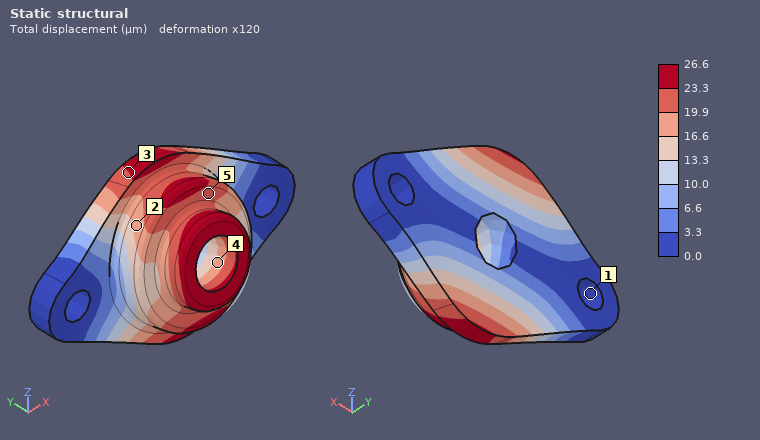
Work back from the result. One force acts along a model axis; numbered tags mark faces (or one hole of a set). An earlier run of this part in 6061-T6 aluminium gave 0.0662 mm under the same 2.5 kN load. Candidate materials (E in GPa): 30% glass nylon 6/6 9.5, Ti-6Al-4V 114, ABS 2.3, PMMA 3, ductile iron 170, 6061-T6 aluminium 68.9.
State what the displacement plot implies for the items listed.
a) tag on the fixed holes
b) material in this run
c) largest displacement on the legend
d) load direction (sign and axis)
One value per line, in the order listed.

1
ductile iron
26.6 µm
+Z
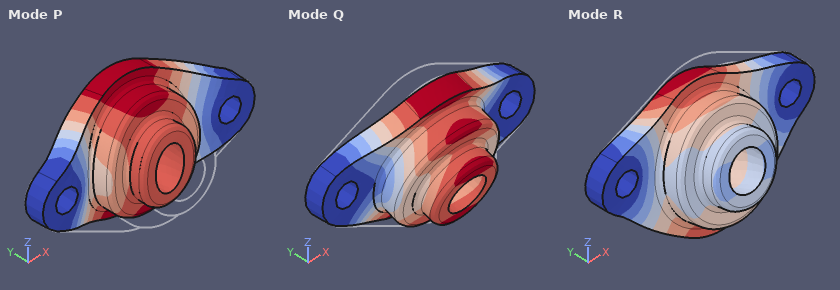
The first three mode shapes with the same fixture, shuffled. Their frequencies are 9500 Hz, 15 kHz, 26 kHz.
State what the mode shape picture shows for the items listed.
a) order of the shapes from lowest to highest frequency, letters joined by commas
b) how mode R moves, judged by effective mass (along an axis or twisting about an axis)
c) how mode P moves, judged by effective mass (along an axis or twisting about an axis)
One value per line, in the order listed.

Q, P, R
along Z
along Y
